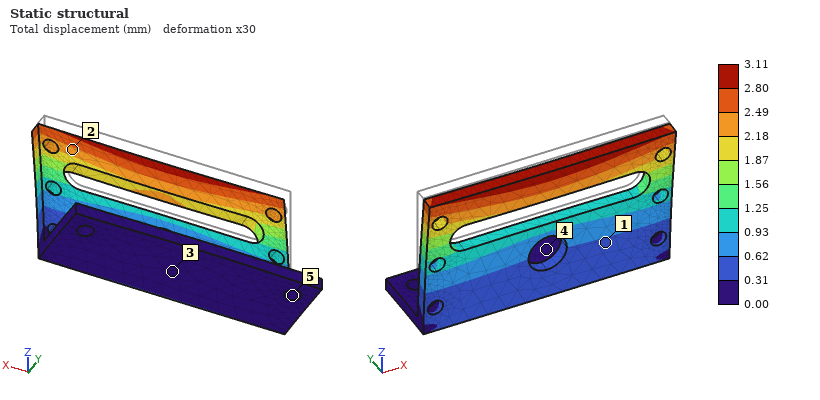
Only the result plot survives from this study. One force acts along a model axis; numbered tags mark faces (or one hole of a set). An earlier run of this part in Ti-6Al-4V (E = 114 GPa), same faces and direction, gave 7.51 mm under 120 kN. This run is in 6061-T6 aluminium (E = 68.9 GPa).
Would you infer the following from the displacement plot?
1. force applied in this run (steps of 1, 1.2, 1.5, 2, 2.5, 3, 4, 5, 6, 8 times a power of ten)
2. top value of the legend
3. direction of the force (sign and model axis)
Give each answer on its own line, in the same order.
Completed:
30 kN
3.11 mm
-Y
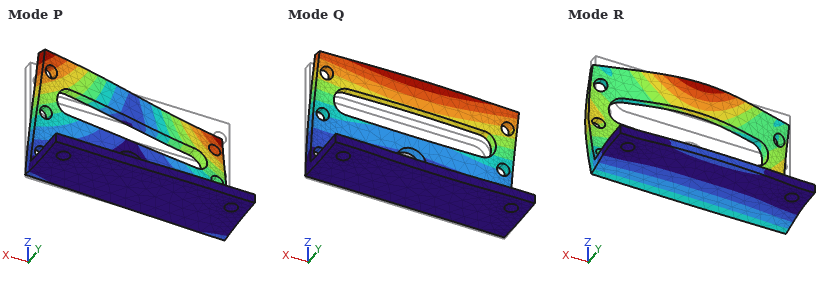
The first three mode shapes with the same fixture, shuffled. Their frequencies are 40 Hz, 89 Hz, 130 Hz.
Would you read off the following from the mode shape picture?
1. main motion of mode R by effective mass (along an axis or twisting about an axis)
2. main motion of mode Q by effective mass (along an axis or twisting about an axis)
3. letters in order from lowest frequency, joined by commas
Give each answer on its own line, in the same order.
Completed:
along Z
along Y
Q, P, R
